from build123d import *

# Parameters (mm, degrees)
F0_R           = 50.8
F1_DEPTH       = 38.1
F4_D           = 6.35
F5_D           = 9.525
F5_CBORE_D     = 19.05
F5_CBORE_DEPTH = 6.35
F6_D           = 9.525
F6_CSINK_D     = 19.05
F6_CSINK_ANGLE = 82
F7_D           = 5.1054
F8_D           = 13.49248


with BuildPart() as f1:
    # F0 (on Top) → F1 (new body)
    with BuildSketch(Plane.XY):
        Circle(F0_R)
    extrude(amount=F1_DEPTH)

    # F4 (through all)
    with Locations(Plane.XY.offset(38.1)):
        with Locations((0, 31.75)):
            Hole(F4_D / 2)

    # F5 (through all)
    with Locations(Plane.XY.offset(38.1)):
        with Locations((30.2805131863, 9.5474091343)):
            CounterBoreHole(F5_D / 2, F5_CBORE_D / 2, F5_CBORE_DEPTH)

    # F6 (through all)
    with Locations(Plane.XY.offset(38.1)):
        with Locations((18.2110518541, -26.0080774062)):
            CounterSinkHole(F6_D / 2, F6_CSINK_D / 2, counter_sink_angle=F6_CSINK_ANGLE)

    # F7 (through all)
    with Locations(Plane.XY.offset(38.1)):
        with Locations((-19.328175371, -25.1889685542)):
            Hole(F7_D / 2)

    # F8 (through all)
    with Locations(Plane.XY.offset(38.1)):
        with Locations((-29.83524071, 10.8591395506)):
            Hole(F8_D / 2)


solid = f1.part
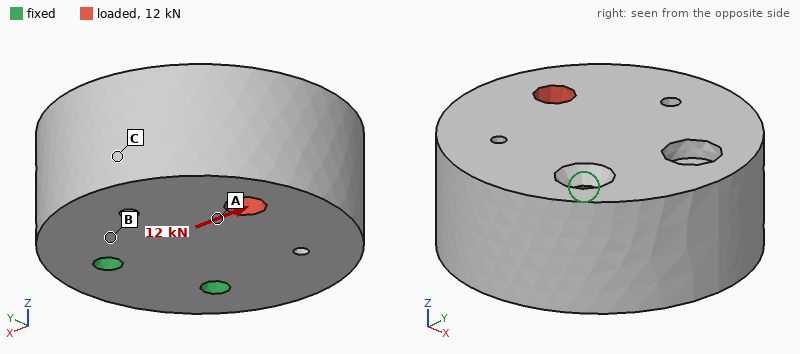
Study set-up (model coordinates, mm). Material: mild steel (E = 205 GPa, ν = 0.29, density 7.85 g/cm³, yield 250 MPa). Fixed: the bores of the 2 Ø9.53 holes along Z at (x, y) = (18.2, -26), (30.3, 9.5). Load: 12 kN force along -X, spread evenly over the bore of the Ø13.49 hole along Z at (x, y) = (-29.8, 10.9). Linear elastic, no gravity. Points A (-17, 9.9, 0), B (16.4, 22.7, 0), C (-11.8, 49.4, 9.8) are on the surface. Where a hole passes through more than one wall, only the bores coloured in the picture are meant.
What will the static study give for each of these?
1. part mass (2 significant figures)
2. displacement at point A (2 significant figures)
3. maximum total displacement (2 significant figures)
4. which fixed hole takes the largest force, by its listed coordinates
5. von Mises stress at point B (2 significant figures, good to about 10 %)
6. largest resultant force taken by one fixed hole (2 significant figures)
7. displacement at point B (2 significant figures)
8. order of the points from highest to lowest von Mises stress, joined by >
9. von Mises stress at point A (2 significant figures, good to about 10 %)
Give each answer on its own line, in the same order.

2.3 kg
2.4 µm
4.0 µm
(30.3, 9.5)
6.0 MPa
11 kN
1.3 µm
A > B > C
8.7 MPa
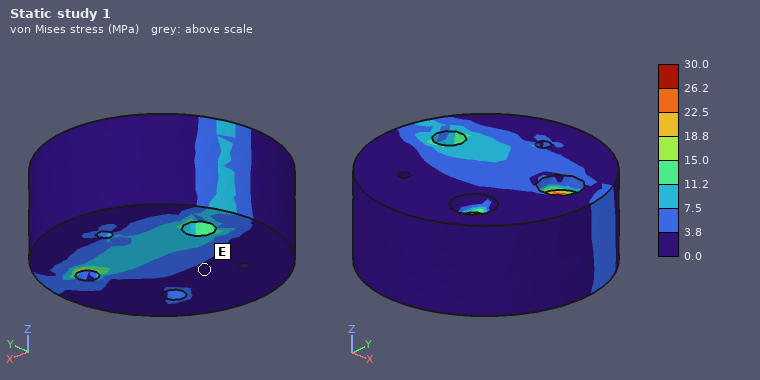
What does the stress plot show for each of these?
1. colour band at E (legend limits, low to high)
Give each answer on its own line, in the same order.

0.0 to 3.8 MPa
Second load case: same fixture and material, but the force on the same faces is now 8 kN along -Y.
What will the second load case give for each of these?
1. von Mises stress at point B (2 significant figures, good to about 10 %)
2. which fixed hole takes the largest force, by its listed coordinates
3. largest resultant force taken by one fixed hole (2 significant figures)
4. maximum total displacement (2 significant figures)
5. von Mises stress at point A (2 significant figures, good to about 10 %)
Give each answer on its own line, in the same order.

4.8 MPa
(18.2, -26)
12 kN
6.1 µm
8.4 MPa
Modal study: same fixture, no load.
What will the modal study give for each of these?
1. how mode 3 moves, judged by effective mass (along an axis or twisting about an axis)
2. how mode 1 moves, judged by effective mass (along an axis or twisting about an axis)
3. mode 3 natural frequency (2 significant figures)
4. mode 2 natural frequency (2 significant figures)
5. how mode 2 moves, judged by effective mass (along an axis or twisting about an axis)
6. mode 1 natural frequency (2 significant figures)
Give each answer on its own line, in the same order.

twisting about X
along Z
8100 Hz
6100 Hz
along Y
4400 Hz
